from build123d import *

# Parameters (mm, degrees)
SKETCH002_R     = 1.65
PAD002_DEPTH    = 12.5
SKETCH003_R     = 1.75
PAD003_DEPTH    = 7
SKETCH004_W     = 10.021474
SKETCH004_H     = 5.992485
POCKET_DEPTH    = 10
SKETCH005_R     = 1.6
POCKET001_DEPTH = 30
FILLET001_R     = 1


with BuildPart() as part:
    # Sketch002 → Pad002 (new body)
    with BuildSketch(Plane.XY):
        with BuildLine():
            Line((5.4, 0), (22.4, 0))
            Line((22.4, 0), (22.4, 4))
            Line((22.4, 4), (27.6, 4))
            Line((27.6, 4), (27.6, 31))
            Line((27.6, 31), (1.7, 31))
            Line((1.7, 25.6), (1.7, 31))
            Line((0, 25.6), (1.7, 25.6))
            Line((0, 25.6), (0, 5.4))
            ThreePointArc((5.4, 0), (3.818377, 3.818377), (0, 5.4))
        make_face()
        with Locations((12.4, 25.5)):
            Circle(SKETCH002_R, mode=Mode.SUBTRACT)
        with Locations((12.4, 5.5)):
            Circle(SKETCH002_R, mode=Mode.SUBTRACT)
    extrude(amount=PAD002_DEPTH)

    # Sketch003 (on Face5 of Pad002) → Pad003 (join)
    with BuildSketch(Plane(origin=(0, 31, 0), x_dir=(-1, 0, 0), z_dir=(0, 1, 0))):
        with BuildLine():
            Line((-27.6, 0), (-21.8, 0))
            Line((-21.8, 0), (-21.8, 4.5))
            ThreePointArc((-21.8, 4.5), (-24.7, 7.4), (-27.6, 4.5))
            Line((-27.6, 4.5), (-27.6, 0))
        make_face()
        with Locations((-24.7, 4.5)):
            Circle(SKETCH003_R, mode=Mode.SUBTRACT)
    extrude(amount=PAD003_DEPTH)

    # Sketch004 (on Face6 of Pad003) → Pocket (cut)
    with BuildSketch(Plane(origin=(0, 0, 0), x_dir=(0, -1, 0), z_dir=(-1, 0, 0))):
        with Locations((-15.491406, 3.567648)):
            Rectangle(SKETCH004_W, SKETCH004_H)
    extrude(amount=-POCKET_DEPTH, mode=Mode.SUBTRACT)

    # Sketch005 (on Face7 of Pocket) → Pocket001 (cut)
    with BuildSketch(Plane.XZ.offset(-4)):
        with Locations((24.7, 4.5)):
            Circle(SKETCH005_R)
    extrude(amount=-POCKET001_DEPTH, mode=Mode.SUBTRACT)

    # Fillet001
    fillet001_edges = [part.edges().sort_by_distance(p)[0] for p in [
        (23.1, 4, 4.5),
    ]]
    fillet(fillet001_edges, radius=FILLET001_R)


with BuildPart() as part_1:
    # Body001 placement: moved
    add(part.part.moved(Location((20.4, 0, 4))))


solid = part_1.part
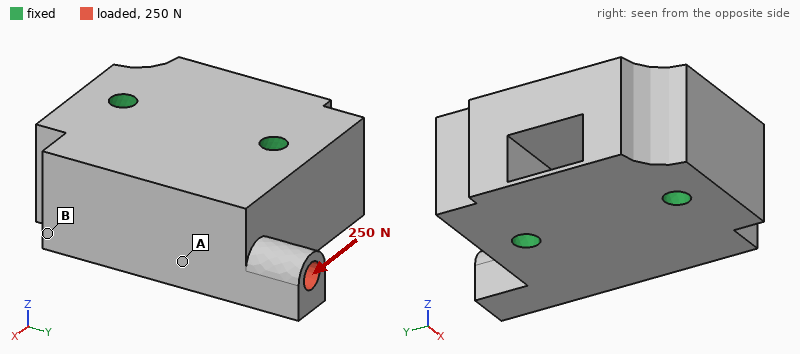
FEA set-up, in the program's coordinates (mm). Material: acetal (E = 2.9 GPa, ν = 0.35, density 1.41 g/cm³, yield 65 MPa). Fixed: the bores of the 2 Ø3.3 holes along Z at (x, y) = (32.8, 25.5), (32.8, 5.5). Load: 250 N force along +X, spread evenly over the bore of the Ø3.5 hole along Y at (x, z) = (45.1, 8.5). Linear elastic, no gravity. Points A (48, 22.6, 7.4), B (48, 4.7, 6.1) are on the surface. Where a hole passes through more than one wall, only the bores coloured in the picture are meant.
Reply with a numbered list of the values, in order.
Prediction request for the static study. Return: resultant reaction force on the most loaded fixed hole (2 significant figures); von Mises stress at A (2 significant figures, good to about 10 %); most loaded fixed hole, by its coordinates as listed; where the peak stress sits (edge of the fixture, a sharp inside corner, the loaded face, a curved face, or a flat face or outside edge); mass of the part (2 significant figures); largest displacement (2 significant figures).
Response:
1. 350 N
2. 7.6 MPa
3. (32.8, 25.5)
4. the loaded face
5. 13 g
6. 0.26 mm
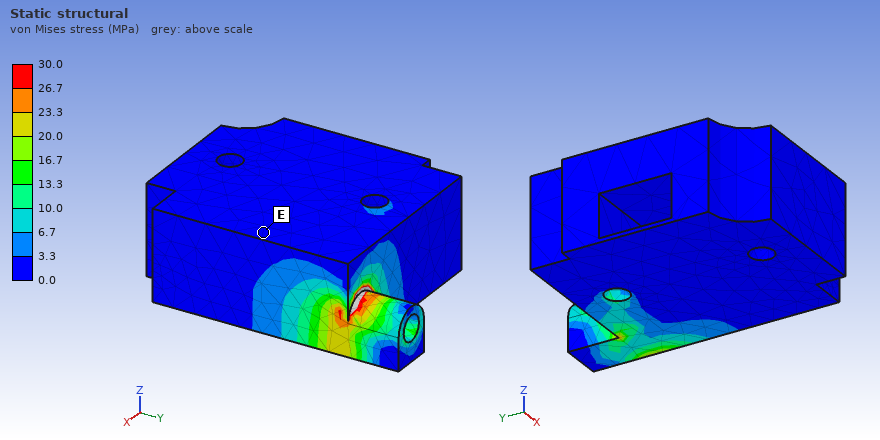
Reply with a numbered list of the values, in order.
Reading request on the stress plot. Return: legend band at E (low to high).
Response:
1. 0.0 to 3.3 MPa
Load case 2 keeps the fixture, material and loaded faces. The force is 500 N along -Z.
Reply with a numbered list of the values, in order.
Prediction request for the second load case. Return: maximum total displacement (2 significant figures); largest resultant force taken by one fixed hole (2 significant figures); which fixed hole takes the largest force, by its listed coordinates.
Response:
1. 0.53 mm
2. 590 N
3. (32.8, 25.5)
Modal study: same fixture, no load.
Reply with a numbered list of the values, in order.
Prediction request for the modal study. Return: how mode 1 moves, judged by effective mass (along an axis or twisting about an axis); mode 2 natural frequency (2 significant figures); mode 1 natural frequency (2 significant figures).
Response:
1. along Z
2. 9700 Hz
3. 7500 Hz
